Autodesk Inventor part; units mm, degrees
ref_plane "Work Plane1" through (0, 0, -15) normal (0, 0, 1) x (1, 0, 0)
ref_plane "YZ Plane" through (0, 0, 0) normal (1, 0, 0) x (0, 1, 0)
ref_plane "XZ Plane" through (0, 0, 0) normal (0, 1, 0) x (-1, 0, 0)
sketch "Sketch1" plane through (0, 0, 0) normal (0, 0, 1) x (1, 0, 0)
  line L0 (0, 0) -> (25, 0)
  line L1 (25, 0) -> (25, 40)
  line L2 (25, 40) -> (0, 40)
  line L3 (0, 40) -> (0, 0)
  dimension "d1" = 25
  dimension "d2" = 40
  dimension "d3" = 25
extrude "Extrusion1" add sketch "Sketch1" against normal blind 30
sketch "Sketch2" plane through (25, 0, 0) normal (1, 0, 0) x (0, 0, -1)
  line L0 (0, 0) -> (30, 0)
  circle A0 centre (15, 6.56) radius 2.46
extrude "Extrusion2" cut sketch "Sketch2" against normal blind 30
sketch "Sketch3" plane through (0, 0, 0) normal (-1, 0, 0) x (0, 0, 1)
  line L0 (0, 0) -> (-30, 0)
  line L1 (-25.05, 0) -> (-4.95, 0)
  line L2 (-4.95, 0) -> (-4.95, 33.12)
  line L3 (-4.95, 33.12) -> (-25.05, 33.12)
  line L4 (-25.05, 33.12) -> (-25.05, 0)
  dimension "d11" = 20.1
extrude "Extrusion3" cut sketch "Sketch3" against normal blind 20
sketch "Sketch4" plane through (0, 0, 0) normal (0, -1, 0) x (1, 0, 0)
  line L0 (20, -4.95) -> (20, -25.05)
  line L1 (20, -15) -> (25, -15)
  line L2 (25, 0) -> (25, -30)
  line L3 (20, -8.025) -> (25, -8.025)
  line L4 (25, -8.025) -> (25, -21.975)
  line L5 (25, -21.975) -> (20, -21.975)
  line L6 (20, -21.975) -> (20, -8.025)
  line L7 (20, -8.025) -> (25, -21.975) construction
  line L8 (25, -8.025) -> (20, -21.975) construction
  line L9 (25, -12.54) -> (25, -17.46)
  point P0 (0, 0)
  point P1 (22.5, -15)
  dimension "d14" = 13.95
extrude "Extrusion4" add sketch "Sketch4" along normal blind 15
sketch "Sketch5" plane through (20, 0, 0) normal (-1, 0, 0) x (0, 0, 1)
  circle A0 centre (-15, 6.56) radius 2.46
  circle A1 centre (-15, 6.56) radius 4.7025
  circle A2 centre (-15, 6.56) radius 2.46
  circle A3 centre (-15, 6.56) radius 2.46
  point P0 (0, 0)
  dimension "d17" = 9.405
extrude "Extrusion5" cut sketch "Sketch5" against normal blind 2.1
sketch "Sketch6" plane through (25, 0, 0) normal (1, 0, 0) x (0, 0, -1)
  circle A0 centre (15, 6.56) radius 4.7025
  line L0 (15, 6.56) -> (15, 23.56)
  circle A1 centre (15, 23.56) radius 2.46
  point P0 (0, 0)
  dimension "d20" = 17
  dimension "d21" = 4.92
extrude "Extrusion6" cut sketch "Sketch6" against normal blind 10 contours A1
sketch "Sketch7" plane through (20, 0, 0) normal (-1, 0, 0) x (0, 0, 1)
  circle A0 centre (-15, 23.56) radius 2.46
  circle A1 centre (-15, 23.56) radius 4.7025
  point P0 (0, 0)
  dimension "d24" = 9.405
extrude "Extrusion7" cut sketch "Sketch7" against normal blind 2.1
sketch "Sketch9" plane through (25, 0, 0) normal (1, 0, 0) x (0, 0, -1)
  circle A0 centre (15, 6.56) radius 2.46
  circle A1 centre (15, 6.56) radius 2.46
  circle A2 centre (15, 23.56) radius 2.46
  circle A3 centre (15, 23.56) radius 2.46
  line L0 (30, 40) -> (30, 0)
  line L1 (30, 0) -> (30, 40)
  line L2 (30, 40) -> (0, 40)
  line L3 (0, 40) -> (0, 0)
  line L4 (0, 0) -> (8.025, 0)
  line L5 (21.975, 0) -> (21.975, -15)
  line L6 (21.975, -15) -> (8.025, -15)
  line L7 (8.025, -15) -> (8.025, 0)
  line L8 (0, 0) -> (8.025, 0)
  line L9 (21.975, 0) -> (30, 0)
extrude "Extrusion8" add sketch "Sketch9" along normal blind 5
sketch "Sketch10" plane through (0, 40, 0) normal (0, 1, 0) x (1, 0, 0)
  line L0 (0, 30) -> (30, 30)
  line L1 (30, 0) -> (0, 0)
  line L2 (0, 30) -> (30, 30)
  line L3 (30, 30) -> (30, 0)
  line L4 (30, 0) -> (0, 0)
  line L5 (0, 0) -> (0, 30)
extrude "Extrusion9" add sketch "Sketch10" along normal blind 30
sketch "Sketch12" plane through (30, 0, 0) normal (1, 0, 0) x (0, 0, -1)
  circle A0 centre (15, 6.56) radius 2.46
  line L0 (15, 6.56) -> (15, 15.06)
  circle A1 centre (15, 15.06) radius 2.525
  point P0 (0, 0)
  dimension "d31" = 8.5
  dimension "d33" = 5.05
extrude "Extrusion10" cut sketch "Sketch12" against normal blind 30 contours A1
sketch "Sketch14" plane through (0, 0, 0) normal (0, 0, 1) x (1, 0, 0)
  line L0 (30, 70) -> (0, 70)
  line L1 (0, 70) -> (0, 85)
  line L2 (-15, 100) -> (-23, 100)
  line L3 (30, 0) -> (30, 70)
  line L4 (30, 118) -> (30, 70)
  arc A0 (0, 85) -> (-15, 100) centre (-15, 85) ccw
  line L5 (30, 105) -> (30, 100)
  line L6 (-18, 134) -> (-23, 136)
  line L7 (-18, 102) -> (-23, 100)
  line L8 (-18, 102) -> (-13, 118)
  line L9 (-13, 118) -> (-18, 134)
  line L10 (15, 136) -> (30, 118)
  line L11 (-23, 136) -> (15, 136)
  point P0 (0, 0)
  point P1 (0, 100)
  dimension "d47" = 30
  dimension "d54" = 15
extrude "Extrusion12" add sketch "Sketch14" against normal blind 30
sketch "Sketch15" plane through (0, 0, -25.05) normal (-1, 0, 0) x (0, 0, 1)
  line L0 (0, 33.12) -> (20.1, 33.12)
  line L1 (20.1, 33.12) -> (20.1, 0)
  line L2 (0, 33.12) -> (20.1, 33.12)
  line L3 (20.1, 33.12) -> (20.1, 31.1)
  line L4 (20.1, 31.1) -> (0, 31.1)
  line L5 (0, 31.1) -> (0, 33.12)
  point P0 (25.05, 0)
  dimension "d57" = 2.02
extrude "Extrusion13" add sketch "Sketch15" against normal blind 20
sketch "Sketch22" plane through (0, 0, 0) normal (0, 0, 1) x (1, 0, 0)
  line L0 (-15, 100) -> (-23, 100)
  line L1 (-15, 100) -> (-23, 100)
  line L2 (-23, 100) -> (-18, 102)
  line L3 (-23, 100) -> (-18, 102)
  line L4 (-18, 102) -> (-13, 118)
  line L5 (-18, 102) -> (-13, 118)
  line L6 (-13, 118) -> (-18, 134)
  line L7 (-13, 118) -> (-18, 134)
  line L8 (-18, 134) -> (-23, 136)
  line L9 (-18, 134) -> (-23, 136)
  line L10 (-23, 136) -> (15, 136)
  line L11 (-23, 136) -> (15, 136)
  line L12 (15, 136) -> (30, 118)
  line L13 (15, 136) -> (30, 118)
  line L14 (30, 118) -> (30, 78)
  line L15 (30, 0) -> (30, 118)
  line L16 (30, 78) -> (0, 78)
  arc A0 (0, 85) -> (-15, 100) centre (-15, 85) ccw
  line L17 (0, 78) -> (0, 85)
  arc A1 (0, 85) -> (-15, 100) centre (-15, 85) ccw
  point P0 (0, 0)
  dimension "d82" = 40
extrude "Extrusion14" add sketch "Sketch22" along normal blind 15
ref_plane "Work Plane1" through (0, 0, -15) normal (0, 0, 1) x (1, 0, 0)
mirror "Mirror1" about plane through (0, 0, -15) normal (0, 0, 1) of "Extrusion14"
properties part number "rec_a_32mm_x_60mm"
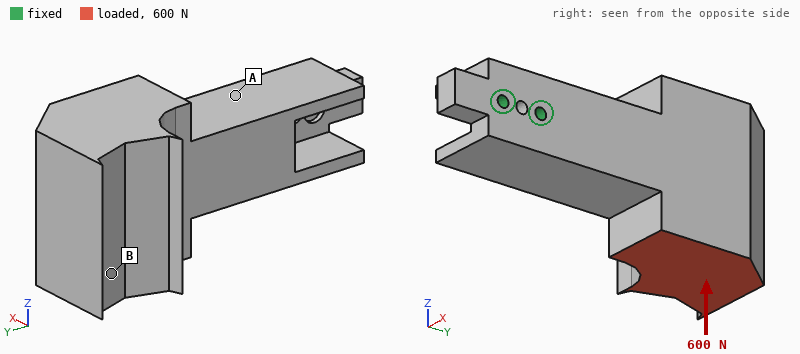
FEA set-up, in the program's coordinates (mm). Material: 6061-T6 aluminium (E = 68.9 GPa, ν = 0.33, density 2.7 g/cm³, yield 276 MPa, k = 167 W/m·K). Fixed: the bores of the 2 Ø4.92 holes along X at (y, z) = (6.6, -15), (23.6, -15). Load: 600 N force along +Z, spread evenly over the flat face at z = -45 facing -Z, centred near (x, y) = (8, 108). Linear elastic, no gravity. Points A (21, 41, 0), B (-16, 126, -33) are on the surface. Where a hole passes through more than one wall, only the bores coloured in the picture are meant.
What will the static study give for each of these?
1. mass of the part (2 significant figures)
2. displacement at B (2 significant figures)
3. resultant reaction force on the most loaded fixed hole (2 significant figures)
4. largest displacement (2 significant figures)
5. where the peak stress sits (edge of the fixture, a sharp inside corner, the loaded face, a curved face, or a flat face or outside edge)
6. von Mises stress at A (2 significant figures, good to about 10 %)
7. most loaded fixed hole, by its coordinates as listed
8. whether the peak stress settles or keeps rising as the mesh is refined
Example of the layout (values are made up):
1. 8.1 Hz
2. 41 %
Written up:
1. 520 g
2. 0.12 mm
3. 2.8 kN
4. 0.13 mm
5. edge of the fixture
6. 12 MPa
7. (23.6, -15)
8. keeps rising
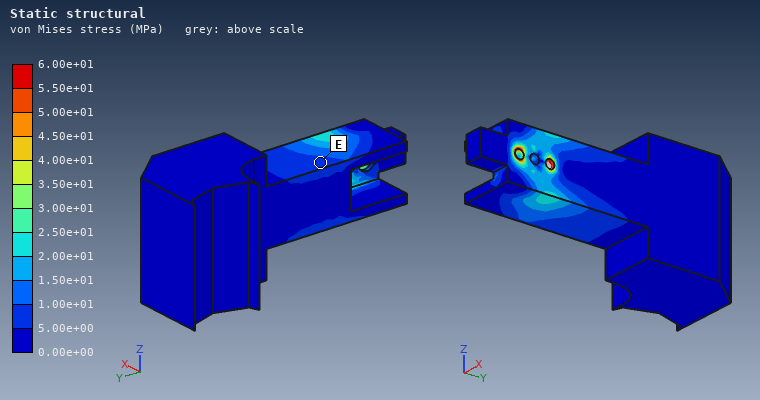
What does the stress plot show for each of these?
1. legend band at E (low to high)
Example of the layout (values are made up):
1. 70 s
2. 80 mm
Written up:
1. 5.00e+00 to 1.00e+01 MPa
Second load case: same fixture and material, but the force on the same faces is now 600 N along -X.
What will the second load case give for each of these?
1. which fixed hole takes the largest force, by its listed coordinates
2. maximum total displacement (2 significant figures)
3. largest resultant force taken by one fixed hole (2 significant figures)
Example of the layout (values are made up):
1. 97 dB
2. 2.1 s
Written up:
1. (23.6, -15)
2. 0.21 mm
3. 2.6 kN
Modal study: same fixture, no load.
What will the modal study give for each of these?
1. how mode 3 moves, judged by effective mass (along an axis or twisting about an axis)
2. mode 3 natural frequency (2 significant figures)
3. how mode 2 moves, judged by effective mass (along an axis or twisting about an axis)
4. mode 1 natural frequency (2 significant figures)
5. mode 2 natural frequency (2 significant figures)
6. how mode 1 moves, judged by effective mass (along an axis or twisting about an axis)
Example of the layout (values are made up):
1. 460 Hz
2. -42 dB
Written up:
1. twisting about Y
2. 1500 Hz
3. along Z
4. 560 Hz
5. 640 Hz
6. along X
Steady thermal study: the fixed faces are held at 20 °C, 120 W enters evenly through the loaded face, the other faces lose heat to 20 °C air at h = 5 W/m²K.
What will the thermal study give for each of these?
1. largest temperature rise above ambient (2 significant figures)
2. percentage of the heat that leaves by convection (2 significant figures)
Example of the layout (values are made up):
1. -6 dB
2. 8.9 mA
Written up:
1. 82 K
2. 5.7 %
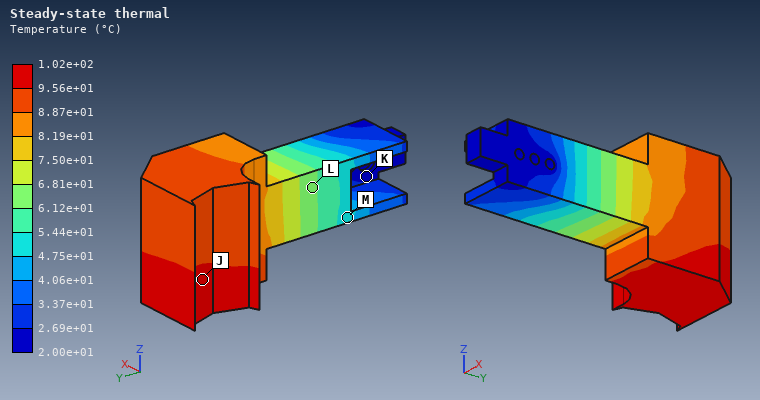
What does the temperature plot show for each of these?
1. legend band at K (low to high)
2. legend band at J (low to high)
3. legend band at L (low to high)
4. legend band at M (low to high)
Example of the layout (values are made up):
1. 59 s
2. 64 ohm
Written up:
1. 2.00e+01 to 2.69e+01 °C
2. 9.56e+01 to 1.02e+02 °C
3. 6.12e+01 to 6.81e+01 °C
4. 4.75e+01 to 5.44e+01 °C
